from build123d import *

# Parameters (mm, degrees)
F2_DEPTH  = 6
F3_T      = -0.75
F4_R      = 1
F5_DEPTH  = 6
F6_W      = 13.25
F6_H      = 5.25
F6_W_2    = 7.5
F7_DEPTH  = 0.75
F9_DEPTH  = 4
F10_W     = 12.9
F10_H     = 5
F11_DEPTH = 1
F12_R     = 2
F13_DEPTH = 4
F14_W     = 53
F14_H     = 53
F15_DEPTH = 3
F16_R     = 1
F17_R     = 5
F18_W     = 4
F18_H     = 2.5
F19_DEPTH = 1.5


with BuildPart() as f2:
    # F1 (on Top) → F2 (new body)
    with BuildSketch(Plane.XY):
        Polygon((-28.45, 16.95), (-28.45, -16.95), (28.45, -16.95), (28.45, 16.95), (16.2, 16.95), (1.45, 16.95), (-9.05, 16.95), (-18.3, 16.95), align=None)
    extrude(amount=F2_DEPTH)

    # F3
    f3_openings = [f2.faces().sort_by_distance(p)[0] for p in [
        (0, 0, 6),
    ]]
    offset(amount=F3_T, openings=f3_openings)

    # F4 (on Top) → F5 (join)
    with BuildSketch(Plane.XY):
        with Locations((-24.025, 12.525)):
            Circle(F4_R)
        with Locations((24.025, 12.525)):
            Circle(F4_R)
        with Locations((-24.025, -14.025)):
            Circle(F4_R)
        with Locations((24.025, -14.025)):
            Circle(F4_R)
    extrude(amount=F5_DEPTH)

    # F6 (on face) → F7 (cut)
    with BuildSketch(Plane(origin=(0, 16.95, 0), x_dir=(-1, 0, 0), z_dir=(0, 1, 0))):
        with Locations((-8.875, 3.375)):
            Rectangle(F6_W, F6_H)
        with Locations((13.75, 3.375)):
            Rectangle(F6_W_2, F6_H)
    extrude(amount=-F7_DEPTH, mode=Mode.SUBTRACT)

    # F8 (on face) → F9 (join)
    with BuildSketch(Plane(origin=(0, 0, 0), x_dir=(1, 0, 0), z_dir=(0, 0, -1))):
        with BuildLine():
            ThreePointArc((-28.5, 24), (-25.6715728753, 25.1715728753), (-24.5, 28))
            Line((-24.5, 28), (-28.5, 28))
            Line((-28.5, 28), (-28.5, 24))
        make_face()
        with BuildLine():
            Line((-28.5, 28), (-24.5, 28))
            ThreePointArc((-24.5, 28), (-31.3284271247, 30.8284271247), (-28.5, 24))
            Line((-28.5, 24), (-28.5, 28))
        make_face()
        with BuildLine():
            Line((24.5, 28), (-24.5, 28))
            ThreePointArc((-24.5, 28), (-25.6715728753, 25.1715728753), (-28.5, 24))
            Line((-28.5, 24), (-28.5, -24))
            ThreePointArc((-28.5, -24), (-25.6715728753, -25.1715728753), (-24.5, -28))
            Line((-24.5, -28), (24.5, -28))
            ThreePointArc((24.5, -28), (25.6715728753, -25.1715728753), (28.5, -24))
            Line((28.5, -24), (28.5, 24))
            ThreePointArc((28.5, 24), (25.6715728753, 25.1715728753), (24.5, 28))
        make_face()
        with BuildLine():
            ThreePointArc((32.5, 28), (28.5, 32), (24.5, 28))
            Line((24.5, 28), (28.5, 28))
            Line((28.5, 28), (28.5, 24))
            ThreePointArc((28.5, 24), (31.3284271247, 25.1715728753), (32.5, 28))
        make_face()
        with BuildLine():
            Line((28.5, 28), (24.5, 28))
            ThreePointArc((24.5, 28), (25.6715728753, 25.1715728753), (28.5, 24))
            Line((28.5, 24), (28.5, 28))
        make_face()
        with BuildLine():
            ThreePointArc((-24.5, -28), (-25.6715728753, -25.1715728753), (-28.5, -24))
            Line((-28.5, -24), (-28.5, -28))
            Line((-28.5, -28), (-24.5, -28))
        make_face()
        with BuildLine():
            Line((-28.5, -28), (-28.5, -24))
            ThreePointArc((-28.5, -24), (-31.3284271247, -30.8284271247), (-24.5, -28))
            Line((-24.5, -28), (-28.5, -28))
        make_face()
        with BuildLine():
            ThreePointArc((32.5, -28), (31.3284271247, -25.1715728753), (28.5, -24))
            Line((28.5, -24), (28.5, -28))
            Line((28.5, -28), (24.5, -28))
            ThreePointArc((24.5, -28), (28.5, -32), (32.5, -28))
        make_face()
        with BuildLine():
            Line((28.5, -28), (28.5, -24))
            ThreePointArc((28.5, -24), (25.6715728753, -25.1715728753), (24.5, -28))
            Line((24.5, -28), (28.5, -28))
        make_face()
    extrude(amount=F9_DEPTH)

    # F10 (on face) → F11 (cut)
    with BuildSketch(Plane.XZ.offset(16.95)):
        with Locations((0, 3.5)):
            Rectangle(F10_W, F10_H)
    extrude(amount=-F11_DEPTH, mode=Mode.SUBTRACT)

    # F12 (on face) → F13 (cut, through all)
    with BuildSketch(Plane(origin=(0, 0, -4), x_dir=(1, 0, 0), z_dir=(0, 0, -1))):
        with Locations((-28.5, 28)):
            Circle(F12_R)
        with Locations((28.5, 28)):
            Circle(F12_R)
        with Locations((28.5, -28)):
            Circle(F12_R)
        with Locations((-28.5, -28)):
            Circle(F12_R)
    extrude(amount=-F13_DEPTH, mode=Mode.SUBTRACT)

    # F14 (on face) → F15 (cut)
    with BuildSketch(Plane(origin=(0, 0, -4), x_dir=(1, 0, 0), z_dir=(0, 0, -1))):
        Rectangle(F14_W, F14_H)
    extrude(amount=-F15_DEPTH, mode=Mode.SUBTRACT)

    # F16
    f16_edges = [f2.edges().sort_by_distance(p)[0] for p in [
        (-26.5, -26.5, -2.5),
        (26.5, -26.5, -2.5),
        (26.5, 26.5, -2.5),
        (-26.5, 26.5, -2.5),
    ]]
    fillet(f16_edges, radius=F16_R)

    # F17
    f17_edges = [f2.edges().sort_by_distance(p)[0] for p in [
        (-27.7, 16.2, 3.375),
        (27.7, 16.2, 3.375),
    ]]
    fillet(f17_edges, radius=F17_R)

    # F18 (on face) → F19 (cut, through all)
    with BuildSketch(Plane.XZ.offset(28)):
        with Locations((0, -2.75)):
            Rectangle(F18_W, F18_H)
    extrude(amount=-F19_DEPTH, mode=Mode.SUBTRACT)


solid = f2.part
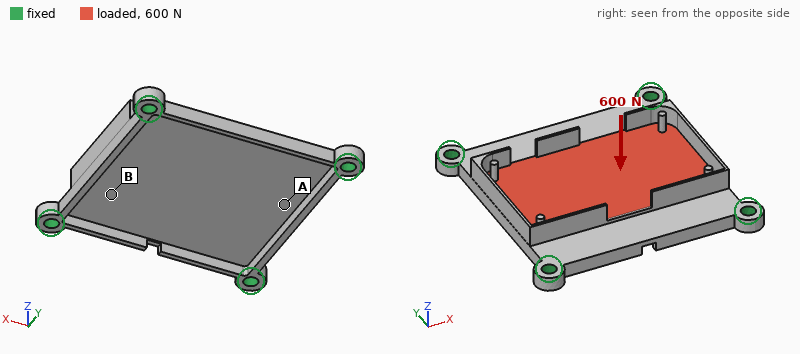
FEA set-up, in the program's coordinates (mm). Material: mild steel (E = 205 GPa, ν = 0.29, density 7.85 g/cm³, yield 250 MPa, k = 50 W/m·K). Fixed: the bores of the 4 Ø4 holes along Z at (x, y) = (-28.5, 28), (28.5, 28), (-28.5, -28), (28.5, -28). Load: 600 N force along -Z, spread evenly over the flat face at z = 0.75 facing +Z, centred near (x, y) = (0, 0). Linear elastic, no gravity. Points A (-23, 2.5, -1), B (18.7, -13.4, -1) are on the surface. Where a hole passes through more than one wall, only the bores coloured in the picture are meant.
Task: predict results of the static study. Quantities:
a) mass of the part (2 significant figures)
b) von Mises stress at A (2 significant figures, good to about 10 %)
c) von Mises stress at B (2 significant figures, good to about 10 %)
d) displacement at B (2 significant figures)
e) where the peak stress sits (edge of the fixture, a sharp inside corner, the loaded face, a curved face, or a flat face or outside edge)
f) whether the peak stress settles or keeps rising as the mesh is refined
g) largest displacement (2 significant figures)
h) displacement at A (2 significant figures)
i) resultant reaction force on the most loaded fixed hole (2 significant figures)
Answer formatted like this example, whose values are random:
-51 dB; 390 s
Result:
54 g; 18 MPa; 47 MPa; 0.043 mm; a sharp inside corner; keeps rising; 0.11 mm; 0.036 mm; 440 N
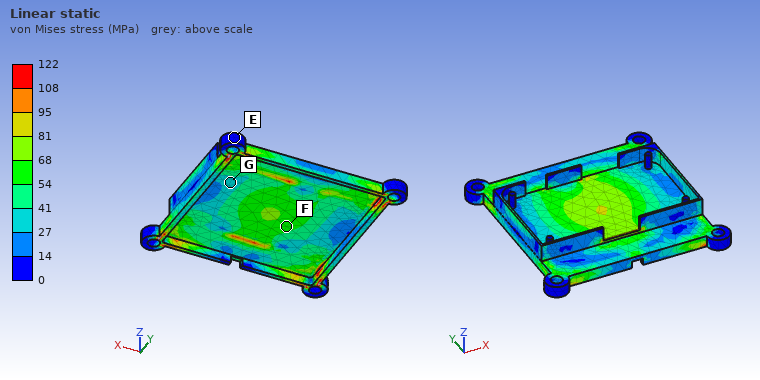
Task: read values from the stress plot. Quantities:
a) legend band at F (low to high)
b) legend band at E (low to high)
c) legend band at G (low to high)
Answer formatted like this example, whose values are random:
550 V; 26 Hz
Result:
54 to 68 MPa; 0 to 14 MPa; 27 to 41 MPa
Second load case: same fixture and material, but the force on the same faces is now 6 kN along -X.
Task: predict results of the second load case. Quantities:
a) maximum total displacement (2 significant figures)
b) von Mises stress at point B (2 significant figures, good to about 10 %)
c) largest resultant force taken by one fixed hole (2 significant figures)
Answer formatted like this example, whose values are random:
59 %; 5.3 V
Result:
19 µm; 49 MPa; 1.7 kN
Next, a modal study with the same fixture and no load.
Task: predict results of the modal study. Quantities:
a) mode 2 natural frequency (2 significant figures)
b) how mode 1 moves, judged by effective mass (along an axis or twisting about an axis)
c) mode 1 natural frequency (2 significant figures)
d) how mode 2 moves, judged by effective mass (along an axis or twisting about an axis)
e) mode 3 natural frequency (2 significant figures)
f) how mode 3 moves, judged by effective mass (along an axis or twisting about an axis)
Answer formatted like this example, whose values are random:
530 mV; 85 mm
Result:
4700 Hz; along Z; 2500 Hz; twisting about X; 6000 Hz; twisting about Y
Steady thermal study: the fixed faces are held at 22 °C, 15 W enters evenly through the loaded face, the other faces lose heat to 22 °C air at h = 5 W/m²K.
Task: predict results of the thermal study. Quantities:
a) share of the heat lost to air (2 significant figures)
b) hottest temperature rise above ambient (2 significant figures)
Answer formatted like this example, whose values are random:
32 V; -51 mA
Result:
10.0 %; 56 K
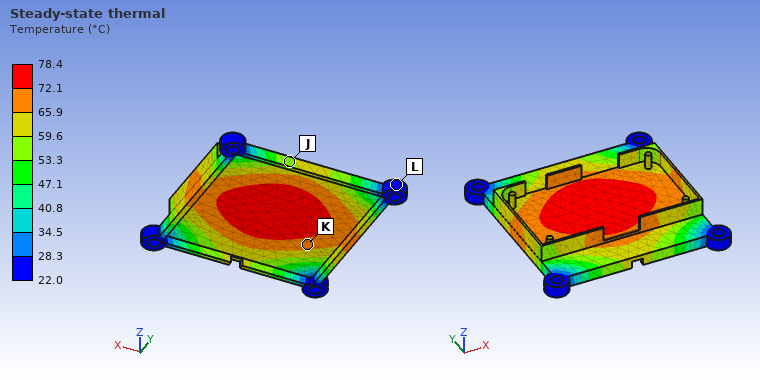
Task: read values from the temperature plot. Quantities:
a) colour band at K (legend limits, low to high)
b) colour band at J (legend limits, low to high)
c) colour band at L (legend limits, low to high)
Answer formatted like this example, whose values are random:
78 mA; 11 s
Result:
65.9 to 72.1 °C; 53.3 to 59.6 °C; 22.0 to 28.3 °C
